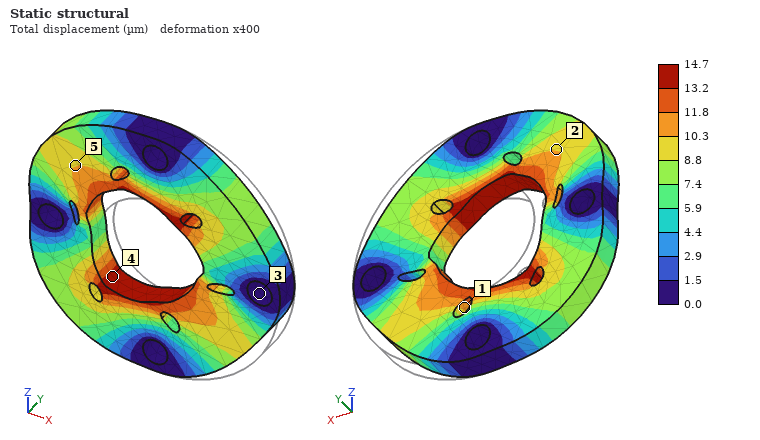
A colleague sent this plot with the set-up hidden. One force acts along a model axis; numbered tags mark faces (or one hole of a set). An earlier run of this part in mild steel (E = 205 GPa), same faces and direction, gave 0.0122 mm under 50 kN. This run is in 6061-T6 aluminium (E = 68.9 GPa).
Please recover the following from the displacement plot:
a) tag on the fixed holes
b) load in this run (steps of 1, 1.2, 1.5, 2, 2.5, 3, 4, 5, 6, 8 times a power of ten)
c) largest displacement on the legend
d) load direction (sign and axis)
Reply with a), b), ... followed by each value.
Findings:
a) 3
b) 20 kN
c) 14.7 µm
d) -X
